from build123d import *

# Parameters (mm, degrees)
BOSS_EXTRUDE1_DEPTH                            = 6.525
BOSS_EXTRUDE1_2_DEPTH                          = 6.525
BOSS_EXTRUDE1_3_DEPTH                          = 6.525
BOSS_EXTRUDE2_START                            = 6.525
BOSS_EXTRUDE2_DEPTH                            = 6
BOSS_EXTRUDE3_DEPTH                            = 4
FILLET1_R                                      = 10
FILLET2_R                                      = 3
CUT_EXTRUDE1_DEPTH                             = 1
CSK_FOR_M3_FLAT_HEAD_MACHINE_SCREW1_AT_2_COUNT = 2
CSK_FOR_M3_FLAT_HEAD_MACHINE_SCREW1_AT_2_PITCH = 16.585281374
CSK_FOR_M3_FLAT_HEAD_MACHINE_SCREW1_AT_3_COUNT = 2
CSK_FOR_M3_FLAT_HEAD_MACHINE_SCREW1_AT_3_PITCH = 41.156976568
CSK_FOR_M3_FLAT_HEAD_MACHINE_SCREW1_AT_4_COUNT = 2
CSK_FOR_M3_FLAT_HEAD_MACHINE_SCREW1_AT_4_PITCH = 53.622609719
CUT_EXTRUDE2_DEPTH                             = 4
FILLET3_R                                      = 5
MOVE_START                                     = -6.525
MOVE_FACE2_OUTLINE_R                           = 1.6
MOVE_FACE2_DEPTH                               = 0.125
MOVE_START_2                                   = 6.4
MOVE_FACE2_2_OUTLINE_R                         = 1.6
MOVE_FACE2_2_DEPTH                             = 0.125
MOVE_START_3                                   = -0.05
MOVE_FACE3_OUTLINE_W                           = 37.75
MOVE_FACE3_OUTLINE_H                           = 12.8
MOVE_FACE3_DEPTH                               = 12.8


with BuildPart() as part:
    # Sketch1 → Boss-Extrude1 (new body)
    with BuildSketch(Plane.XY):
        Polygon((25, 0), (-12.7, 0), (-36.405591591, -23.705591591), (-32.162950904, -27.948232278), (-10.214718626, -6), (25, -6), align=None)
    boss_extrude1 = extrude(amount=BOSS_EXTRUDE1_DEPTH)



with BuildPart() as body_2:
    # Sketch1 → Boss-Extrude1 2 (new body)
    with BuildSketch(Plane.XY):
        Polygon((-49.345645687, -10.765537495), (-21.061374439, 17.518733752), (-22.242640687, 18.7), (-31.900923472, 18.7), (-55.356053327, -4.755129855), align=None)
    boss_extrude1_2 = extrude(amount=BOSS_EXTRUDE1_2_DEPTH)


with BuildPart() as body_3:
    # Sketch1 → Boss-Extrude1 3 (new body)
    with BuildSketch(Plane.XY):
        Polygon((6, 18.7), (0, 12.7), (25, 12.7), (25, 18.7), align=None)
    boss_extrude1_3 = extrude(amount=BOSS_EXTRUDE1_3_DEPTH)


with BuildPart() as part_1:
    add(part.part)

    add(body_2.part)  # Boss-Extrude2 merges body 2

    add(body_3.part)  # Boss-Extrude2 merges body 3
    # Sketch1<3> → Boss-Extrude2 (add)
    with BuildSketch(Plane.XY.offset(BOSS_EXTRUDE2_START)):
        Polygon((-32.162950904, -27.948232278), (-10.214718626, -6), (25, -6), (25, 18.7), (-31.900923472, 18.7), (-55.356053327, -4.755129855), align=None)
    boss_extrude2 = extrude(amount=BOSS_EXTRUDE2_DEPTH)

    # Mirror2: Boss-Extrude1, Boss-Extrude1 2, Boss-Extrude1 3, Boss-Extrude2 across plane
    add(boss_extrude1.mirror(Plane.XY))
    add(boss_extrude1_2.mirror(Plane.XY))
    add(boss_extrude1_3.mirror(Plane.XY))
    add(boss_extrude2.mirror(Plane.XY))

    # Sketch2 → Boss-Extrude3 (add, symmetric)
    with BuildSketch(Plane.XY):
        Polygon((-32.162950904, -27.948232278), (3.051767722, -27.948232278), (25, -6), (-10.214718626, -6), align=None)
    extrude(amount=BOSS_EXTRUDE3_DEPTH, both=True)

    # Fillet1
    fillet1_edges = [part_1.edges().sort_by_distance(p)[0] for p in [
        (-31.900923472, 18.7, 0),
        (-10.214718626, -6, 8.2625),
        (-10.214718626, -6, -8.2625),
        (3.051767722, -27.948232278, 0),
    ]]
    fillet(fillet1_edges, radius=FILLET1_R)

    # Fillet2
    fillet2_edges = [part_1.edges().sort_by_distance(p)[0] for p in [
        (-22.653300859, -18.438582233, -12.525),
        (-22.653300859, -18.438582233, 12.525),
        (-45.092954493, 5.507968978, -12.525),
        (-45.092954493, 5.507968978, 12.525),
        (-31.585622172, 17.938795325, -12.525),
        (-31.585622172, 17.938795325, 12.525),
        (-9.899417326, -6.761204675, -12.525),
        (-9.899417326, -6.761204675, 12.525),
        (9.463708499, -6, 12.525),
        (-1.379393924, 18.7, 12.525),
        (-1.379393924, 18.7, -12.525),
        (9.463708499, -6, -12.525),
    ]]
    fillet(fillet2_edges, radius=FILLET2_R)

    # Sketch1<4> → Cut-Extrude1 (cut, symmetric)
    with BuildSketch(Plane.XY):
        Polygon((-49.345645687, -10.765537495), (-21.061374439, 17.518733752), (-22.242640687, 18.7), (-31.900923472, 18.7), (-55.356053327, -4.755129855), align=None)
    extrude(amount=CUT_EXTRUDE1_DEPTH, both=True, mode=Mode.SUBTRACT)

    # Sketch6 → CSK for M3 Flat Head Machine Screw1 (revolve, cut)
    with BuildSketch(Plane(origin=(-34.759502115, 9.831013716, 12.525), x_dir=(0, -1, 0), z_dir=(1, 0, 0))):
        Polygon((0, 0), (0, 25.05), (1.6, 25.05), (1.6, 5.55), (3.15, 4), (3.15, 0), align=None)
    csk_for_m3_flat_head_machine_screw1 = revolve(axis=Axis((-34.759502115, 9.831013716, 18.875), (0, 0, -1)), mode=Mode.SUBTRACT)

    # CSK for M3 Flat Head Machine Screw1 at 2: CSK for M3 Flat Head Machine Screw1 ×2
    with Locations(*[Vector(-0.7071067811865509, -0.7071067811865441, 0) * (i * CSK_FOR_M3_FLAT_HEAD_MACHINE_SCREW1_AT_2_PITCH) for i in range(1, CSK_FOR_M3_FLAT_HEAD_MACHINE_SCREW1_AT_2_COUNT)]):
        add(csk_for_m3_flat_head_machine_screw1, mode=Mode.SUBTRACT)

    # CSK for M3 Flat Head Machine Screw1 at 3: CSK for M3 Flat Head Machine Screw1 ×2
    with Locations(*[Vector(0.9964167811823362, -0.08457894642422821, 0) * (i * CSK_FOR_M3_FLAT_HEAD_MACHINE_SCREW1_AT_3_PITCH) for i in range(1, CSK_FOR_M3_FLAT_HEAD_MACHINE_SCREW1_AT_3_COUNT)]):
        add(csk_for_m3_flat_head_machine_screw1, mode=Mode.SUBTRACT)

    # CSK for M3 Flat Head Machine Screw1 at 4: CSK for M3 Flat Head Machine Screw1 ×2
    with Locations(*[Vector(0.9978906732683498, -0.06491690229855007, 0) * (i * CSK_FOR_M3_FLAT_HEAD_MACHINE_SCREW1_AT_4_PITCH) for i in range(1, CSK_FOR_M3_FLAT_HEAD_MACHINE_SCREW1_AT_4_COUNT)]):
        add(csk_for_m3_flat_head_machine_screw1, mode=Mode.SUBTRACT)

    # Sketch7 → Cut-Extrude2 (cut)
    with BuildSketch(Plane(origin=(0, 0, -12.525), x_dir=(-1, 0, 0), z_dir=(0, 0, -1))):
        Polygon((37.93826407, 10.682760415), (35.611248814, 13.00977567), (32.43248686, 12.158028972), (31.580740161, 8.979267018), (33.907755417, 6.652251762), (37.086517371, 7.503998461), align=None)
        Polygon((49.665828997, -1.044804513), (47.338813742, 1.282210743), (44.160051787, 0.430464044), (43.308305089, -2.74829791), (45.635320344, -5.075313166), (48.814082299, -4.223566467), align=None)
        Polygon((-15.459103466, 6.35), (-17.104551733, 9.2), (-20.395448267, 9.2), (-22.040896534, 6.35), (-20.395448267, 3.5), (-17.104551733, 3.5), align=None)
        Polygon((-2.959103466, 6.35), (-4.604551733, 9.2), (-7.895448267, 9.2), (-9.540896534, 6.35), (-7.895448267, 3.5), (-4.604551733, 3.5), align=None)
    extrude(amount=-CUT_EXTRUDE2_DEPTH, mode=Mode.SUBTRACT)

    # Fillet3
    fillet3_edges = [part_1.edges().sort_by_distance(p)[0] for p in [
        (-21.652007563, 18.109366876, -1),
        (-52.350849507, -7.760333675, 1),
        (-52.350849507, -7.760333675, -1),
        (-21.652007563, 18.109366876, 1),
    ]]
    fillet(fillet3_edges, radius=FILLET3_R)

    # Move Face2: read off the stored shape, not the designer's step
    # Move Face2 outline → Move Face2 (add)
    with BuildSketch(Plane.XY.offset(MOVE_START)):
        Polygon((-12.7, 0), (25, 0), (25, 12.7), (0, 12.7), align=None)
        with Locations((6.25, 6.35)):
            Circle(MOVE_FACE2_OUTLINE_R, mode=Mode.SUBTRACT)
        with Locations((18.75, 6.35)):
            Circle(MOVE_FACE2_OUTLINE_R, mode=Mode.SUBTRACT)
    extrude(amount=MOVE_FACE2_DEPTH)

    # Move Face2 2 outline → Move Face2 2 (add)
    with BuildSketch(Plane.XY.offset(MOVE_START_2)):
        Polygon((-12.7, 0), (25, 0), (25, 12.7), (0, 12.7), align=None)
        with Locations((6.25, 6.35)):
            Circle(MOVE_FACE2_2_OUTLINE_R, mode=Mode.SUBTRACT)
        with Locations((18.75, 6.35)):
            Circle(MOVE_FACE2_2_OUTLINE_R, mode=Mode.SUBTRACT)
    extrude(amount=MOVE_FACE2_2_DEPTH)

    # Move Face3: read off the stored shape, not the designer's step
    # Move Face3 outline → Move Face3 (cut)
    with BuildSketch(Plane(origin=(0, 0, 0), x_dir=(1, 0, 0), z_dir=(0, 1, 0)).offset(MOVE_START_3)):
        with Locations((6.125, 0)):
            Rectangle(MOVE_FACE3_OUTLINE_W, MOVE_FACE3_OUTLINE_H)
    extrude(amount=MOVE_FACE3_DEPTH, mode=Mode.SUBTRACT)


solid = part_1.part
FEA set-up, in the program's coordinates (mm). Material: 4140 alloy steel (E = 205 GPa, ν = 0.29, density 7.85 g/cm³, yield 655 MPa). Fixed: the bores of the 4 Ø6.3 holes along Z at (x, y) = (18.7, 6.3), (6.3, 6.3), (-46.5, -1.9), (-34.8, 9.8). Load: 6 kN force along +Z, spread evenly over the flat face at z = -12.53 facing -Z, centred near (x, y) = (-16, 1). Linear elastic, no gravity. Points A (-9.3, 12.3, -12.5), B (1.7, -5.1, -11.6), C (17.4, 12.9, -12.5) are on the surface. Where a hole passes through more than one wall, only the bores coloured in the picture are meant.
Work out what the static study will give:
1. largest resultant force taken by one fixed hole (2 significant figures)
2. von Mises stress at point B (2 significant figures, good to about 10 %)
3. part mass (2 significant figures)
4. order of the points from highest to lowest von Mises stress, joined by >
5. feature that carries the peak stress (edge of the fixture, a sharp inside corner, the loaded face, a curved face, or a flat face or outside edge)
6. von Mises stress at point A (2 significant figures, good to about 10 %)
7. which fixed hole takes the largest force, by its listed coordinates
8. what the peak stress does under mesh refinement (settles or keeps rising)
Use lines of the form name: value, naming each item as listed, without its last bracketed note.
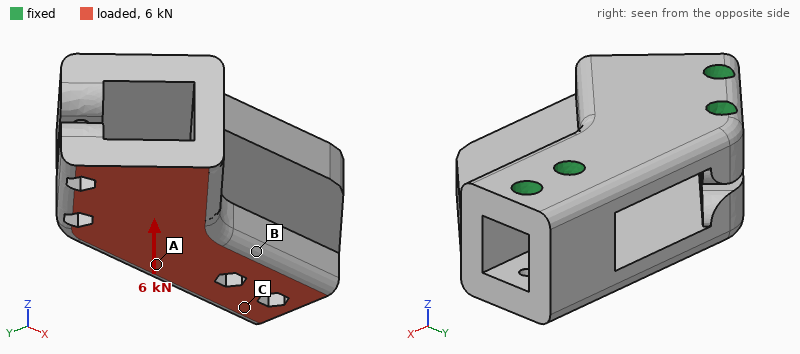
largest resultant force taken by one fixed hole: 5.1 kN
von Mises stress at point B: 43 MPa
part mass: 320 g
order of the points from highest to lowest von Mises stress, joined by >: A > B > C
feature that carries the peak stress: edge of the fixture
von Mises stress at point A: 86 MPa
which fixed hole takes the largest force, by its listed coordinates: (6.3, 6.3)
what the peak stress does under mesh refinement: keeps rising
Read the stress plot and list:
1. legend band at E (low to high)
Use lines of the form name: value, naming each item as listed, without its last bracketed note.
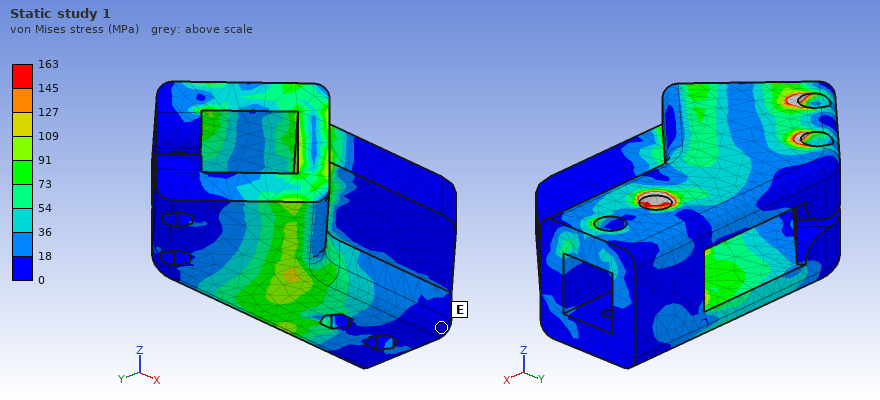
legend band at E: 0 to 18 MPa
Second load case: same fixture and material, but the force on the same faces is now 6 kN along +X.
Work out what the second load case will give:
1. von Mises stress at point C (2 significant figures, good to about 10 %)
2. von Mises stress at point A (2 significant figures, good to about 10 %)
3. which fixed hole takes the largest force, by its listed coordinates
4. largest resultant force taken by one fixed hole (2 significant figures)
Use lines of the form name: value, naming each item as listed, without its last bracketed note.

von Mises stress at point C: 12 MPa
von Mises stress at point A: 30 MPa
which fixed hole takes the largest force, by its listed coordinates: (18.7, 6.3)
largest resultant force taken by one fixed hole: 4.7 kN
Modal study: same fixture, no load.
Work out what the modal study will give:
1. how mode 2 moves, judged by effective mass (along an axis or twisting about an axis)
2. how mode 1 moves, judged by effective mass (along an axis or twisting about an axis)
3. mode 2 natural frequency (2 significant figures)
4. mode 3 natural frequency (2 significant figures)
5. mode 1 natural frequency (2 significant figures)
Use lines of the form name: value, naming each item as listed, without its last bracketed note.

how mode 2 moves, judged by effective mass: along Z
how mode 1 moves, judged by effective mass: along Y
mode 2 natural frequency: 3300 Hz
mode 3 natural frequency: 6900 Hz
mode 1 natural frequency: 3100 Hz
